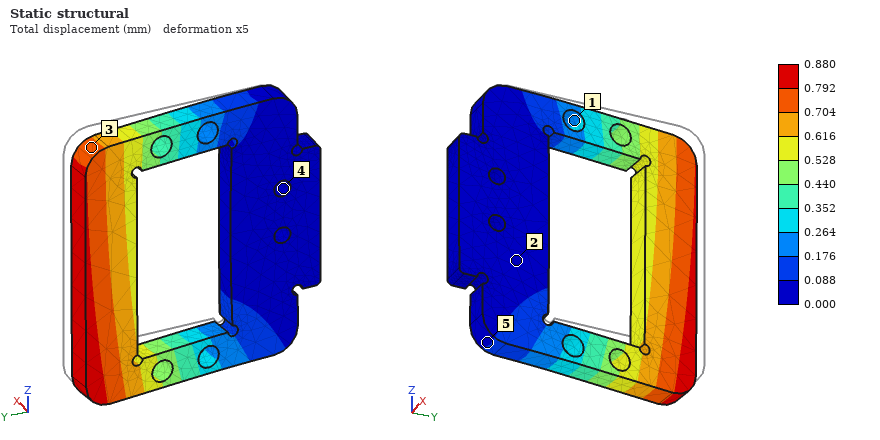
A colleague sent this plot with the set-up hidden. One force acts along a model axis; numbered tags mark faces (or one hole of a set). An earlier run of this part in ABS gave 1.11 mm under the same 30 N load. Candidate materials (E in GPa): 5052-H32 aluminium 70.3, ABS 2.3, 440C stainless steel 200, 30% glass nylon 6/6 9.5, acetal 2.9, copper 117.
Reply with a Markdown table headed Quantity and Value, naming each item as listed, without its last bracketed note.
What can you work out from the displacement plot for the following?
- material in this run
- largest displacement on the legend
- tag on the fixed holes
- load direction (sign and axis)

| Quantity | Value |
|---|---|
| material in this run | acetal |
| largest displacement on the legend | 0.880 mm |
| tag on the fixed holes | 4 |
| load direction | -X |
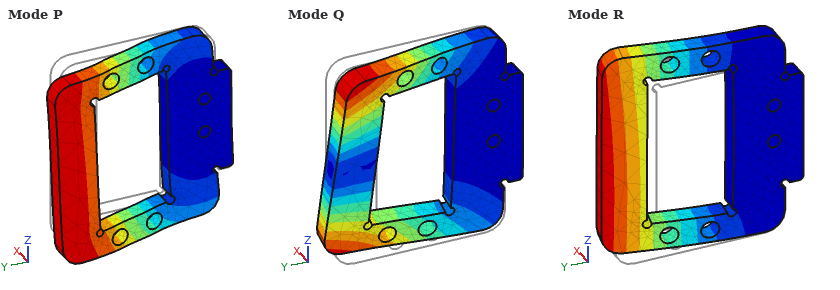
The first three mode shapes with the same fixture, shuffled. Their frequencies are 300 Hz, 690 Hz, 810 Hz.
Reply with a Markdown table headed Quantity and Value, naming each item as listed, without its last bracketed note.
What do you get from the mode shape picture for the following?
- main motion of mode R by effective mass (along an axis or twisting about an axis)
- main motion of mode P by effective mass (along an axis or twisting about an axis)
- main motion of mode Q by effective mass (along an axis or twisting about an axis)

| Quantity | Value |
|---|---|
| main motion of mode R by effective mass | along X |
| main motion of mode P by effective mass | along Z |
| main motion of mode Q by effective mass | twisting about Y |
